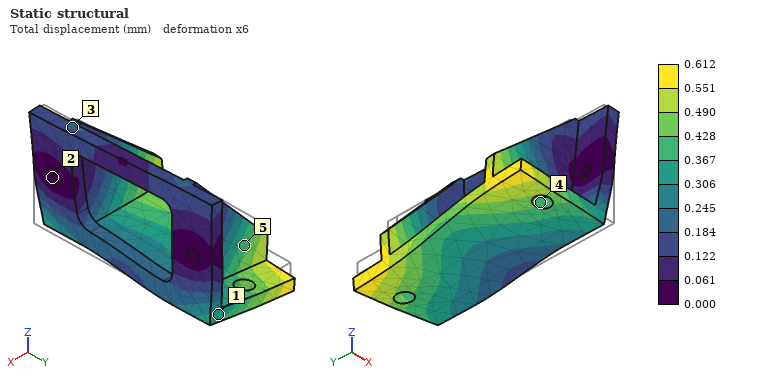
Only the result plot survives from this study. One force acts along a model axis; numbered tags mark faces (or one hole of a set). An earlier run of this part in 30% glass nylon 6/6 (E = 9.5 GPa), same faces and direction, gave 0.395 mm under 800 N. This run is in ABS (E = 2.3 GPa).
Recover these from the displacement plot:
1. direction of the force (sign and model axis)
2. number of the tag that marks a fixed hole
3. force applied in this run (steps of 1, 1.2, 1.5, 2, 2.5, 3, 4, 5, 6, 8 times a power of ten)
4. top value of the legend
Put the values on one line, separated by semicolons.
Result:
+Y; 2; 300 N; 0.612 mm
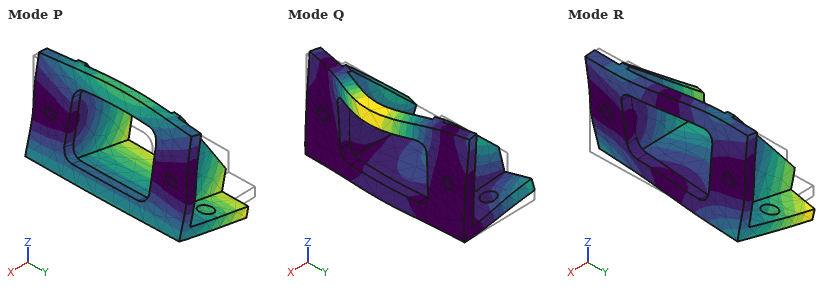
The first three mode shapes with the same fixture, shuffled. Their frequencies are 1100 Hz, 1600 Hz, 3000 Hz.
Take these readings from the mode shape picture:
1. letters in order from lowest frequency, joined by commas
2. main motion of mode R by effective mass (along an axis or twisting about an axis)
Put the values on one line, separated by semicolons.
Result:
P, R, Q; along Y
